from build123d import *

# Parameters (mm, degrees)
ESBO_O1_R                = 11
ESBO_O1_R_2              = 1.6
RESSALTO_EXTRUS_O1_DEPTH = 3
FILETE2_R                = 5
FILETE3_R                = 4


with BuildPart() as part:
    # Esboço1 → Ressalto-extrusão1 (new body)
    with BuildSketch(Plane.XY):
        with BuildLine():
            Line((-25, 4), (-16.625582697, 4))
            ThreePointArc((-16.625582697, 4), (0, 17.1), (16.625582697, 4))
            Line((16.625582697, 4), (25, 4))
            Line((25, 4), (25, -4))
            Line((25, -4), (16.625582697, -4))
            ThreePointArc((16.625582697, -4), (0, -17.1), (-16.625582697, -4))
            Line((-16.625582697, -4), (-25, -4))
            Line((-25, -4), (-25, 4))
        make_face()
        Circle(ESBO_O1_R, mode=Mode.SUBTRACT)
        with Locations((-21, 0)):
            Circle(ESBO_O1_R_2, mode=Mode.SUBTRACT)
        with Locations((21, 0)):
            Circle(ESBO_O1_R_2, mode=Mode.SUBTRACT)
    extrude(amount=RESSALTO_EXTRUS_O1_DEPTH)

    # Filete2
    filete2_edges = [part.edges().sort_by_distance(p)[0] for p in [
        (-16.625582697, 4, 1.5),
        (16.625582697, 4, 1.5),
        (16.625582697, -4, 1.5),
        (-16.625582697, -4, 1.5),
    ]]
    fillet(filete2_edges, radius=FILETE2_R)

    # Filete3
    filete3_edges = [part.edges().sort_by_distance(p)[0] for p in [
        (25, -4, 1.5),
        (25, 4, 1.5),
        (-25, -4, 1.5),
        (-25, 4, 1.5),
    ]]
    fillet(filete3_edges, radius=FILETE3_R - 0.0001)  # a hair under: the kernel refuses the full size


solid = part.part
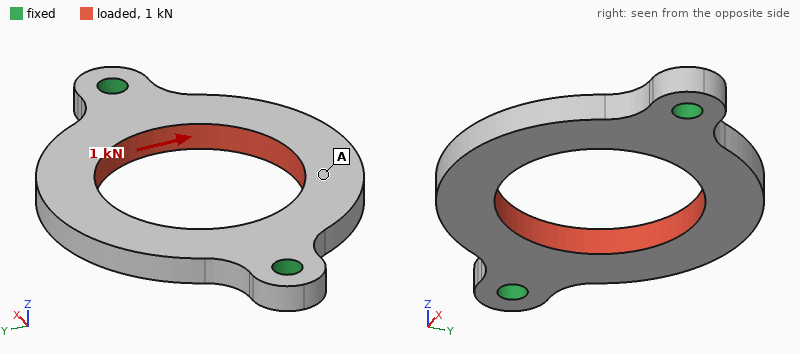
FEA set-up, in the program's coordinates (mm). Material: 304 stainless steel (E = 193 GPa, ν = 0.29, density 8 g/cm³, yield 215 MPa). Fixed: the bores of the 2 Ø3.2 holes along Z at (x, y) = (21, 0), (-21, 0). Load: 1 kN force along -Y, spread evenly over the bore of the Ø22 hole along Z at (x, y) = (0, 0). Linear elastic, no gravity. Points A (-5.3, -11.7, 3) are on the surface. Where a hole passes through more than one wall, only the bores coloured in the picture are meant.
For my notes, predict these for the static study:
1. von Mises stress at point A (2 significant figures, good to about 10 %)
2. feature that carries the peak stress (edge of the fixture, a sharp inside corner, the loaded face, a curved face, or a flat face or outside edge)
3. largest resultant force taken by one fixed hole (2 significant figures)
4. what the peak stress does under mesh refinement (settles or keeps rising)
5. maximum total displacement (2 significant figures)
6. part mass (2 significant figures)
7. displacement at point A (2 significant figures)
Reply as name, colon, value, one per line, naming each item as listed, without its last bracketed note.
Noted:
von Mises stress at point A: 14 MPa
feature that carries the peak stress: edge of the fixture
largest resultant force taken by one fixed hole: 500 N
what the peak stress does under mesh refinement: keeps rising
maximum total displacement: 3.3 µm
part mass: 16 g
displacement at point A: 3.2 µm
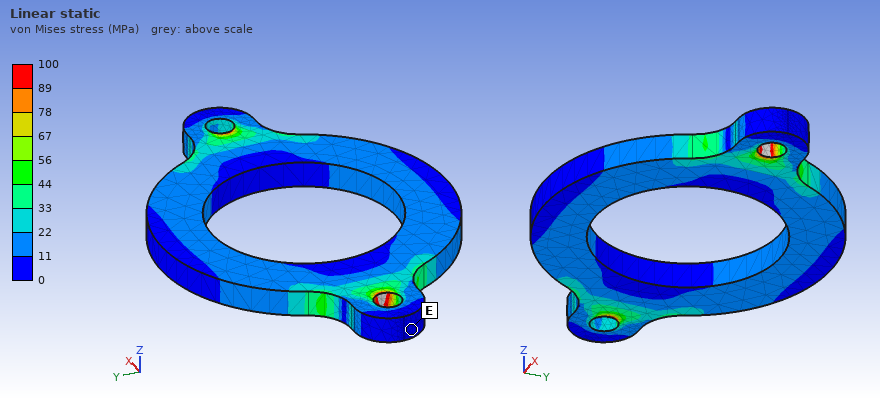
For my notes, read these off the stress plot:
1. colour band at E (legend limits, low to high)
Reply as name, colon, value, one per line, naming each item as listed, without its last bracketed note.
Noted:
colour band at E: 0 to 11 MPa
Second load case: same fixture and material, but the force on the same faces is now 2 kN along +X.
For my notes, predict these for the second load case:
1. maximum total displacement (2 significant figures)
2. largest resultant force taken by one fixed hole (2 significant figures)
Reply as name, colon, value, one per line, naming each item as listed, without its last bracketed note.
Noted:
maximum total displacement: 5.5 µm
largest resultant force taken by one fixed hole: 1.0 kN
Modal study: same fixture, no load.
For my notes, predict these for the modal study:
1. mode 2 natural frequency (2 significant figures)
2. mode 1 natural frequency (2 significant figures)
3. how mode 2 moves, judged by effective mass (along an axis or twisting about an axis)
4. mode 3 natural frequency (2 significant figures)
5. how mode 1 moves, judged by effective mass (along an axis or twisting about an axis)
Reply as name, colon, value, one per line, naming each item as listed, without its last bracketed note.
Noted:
mode 2 natural frequency: 5600 Hz
mode 1 natural frequency: 4700 Hz
how mode 2 moves, judged by effective mass: along Z
mode 3 natural frequency: 14 kHz
how mode 1 moves, judged by effective mass: twisting about X
